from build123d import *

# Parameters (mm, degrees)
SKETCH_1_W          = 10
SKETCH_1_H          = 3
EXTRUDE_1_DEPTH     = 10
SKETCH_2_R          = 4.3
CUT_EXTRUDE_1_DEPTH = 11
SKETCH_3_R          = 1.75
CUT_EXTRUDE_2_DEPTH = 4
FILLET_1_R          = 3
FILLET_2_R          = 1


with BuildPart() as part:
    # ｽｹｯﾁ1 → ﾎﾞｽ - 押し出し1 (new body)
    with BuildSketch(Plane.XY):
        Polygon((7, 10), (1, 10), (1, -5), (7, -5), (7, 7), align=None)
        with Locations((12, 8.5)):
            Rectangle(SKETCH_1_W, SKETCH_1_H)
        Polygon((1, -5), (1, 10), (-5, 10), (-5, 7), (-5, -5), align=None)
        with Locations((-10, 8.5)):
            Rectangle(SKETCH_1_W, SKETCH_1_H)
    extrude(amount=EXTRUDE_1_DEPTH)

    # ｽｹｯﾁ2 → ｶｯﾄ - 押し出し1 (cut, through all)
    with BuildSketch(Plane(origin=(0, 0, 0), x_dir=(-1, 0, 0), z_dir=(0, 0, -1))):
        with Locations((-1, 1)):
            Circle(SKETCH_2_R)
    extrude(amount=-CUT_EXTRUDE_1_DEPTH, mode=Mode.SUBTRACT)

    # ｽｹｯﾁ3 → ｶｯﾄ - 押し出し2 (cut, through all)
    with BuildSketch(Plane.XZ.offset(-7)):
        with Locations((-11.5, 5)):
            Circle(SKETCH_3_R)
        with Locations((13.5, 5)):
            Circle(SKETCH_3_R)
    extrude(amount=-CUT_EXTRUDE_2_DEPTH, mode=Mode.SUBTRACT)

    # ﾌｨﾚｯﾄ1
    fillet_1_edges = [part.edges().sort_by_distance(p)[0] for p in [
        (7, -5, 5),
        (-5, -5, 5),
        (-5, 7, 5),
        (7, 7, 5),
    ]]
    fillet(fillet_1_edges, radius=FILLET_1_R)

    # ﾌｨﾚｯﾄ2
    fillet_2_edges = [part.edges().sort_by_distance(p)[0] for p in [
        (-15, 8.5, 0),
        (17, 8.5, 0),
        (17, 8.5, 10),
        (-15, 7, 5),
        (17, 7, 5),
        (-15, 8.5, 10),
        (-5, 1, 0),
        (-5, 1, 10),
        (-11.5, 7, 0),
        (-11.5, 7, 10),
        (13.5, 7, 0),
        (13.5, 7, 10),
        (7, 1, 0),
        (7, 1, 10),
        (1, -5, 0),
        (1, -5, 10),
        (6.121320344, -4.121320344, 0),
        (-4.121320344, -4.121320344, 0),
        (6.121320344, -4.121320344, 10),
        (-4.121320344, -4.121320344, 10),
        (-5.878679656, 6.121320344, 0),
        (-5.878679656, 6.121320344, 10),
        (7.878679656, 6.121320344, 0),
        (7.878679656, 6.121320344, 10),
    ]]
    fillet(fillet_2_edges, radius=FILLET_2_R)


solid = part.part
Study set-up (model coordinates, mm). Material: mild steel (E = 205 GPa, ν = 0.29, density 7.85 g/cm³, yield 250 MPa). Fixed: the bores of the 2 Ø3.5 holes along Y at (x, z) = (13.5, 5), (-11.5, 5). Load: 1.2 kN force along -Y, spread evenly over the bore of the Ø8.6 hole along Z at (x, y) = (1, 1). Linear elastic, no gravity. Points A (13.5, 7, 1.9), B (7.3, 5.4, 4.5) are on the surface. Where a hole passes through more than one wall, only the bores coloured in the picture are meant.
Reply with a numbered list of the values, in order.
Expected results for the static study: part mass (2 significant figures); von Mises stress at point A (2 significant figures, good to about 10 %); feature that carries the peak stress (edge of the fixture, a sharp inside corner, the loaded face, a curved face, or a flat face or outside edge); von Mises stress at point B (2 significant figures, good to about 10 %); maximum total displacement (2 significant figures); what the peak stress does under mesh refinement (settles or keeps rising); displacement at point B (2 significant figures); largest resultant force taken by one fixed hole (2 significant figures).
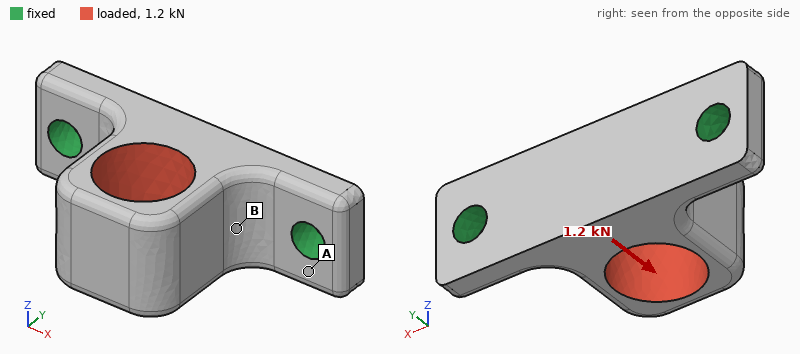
1. 14 g
2. 33 MPa
3. edge of the fixture
4. 77 MPa
5. 6.0 µm
6. keeps rising
7. 4.4 µm
8. 690 N
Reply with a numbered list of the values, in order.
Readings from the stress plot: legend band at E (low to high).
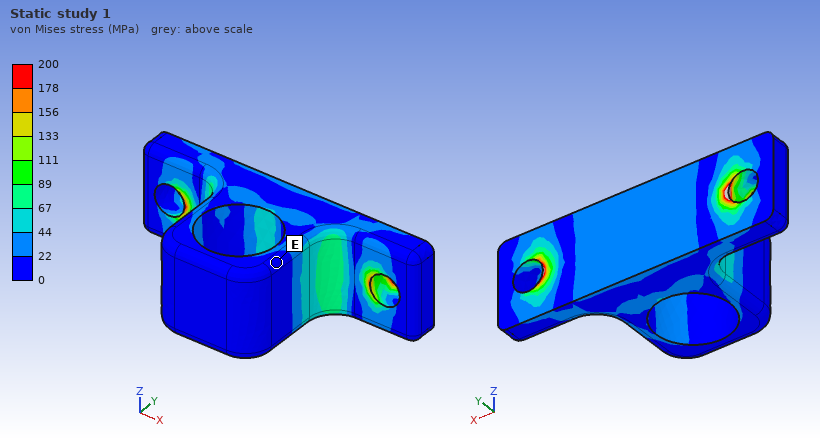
1. 0 to 22 MPa
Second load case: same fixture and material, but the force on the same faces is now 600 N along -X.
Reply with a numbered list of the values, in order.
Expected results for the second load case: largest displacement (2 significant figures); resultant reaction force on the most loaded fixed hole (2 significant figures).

1. 6.9 µm
2. 380 N
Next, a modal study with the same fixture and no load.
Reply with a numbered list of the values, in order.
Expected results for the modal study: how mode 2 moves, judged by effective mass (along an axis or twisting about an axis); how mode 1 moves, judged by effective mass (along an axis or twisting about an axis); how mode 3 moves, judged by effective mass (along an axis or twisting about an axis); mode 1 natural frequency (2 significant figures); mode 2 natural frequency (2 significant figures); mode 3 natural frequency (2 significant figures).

1. along X
2. along Z
3. along Y
4. 11 kHz
5. 21 kHz
6. 23 kHz
